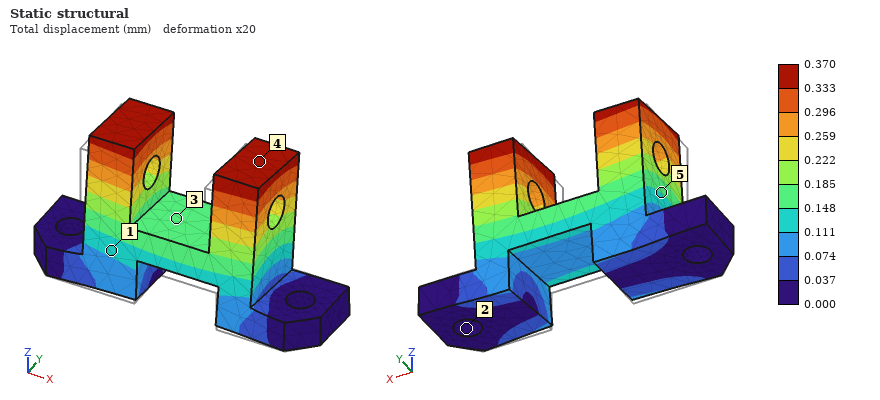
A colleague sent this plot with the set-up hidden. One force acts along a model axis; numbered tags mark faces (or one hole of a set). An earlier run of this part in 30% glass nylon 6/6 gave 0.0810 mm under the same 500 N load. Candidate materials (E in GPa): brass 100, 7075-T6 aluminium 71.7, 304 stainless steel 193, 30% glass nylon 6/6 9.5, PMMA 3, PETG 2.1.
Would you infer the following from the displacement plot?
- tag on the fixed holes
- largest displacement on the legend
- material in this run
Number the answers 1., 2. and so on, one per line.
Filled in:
1. 2
2. 0.370 mm
3. PETG
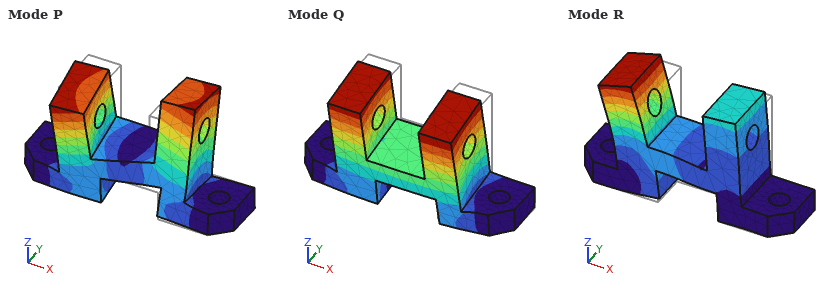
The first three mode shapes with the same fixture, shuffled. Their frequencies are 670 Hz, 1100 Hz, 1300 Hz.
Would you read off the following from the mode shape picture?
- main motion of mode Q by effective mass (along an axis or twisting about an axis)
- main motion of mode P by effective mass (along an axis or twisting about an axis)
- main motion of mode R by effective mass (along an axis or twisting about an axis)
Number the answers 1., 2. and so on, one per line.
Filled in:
1. along Y
2. twisting about Z
3. along X
